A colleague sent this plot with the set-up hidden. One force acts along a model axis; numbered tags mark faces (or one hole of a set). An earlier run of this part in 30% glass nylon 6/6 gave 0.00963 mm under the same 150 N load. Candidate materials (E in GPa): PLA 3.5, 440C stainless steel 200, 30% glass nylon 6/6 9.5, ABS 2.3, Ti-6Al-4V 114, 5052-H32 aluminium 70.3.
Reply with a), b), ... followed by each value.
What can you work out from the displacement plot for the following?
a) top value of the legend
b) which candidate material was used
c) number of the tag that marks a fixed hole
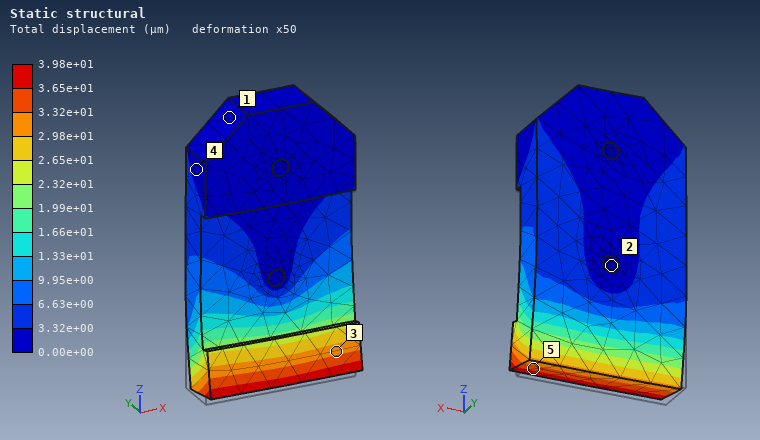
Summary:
a) 3.98e+01 µm
b) ABS
c) 2
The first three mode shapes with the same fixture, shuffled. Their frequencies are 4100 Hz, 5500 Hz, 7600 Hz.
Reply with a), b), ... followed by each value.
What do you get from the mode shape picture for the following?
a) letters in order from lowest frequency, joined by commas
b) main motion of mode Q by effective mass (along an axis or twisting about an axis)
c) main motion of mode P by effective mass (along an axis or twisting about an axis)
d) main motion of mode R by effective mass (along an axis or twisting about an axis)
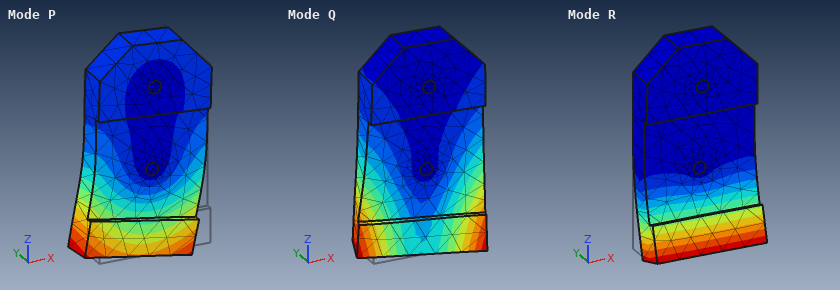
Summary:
a) R, Q, P
b) twisting about Z
c) along X
d) along Y
